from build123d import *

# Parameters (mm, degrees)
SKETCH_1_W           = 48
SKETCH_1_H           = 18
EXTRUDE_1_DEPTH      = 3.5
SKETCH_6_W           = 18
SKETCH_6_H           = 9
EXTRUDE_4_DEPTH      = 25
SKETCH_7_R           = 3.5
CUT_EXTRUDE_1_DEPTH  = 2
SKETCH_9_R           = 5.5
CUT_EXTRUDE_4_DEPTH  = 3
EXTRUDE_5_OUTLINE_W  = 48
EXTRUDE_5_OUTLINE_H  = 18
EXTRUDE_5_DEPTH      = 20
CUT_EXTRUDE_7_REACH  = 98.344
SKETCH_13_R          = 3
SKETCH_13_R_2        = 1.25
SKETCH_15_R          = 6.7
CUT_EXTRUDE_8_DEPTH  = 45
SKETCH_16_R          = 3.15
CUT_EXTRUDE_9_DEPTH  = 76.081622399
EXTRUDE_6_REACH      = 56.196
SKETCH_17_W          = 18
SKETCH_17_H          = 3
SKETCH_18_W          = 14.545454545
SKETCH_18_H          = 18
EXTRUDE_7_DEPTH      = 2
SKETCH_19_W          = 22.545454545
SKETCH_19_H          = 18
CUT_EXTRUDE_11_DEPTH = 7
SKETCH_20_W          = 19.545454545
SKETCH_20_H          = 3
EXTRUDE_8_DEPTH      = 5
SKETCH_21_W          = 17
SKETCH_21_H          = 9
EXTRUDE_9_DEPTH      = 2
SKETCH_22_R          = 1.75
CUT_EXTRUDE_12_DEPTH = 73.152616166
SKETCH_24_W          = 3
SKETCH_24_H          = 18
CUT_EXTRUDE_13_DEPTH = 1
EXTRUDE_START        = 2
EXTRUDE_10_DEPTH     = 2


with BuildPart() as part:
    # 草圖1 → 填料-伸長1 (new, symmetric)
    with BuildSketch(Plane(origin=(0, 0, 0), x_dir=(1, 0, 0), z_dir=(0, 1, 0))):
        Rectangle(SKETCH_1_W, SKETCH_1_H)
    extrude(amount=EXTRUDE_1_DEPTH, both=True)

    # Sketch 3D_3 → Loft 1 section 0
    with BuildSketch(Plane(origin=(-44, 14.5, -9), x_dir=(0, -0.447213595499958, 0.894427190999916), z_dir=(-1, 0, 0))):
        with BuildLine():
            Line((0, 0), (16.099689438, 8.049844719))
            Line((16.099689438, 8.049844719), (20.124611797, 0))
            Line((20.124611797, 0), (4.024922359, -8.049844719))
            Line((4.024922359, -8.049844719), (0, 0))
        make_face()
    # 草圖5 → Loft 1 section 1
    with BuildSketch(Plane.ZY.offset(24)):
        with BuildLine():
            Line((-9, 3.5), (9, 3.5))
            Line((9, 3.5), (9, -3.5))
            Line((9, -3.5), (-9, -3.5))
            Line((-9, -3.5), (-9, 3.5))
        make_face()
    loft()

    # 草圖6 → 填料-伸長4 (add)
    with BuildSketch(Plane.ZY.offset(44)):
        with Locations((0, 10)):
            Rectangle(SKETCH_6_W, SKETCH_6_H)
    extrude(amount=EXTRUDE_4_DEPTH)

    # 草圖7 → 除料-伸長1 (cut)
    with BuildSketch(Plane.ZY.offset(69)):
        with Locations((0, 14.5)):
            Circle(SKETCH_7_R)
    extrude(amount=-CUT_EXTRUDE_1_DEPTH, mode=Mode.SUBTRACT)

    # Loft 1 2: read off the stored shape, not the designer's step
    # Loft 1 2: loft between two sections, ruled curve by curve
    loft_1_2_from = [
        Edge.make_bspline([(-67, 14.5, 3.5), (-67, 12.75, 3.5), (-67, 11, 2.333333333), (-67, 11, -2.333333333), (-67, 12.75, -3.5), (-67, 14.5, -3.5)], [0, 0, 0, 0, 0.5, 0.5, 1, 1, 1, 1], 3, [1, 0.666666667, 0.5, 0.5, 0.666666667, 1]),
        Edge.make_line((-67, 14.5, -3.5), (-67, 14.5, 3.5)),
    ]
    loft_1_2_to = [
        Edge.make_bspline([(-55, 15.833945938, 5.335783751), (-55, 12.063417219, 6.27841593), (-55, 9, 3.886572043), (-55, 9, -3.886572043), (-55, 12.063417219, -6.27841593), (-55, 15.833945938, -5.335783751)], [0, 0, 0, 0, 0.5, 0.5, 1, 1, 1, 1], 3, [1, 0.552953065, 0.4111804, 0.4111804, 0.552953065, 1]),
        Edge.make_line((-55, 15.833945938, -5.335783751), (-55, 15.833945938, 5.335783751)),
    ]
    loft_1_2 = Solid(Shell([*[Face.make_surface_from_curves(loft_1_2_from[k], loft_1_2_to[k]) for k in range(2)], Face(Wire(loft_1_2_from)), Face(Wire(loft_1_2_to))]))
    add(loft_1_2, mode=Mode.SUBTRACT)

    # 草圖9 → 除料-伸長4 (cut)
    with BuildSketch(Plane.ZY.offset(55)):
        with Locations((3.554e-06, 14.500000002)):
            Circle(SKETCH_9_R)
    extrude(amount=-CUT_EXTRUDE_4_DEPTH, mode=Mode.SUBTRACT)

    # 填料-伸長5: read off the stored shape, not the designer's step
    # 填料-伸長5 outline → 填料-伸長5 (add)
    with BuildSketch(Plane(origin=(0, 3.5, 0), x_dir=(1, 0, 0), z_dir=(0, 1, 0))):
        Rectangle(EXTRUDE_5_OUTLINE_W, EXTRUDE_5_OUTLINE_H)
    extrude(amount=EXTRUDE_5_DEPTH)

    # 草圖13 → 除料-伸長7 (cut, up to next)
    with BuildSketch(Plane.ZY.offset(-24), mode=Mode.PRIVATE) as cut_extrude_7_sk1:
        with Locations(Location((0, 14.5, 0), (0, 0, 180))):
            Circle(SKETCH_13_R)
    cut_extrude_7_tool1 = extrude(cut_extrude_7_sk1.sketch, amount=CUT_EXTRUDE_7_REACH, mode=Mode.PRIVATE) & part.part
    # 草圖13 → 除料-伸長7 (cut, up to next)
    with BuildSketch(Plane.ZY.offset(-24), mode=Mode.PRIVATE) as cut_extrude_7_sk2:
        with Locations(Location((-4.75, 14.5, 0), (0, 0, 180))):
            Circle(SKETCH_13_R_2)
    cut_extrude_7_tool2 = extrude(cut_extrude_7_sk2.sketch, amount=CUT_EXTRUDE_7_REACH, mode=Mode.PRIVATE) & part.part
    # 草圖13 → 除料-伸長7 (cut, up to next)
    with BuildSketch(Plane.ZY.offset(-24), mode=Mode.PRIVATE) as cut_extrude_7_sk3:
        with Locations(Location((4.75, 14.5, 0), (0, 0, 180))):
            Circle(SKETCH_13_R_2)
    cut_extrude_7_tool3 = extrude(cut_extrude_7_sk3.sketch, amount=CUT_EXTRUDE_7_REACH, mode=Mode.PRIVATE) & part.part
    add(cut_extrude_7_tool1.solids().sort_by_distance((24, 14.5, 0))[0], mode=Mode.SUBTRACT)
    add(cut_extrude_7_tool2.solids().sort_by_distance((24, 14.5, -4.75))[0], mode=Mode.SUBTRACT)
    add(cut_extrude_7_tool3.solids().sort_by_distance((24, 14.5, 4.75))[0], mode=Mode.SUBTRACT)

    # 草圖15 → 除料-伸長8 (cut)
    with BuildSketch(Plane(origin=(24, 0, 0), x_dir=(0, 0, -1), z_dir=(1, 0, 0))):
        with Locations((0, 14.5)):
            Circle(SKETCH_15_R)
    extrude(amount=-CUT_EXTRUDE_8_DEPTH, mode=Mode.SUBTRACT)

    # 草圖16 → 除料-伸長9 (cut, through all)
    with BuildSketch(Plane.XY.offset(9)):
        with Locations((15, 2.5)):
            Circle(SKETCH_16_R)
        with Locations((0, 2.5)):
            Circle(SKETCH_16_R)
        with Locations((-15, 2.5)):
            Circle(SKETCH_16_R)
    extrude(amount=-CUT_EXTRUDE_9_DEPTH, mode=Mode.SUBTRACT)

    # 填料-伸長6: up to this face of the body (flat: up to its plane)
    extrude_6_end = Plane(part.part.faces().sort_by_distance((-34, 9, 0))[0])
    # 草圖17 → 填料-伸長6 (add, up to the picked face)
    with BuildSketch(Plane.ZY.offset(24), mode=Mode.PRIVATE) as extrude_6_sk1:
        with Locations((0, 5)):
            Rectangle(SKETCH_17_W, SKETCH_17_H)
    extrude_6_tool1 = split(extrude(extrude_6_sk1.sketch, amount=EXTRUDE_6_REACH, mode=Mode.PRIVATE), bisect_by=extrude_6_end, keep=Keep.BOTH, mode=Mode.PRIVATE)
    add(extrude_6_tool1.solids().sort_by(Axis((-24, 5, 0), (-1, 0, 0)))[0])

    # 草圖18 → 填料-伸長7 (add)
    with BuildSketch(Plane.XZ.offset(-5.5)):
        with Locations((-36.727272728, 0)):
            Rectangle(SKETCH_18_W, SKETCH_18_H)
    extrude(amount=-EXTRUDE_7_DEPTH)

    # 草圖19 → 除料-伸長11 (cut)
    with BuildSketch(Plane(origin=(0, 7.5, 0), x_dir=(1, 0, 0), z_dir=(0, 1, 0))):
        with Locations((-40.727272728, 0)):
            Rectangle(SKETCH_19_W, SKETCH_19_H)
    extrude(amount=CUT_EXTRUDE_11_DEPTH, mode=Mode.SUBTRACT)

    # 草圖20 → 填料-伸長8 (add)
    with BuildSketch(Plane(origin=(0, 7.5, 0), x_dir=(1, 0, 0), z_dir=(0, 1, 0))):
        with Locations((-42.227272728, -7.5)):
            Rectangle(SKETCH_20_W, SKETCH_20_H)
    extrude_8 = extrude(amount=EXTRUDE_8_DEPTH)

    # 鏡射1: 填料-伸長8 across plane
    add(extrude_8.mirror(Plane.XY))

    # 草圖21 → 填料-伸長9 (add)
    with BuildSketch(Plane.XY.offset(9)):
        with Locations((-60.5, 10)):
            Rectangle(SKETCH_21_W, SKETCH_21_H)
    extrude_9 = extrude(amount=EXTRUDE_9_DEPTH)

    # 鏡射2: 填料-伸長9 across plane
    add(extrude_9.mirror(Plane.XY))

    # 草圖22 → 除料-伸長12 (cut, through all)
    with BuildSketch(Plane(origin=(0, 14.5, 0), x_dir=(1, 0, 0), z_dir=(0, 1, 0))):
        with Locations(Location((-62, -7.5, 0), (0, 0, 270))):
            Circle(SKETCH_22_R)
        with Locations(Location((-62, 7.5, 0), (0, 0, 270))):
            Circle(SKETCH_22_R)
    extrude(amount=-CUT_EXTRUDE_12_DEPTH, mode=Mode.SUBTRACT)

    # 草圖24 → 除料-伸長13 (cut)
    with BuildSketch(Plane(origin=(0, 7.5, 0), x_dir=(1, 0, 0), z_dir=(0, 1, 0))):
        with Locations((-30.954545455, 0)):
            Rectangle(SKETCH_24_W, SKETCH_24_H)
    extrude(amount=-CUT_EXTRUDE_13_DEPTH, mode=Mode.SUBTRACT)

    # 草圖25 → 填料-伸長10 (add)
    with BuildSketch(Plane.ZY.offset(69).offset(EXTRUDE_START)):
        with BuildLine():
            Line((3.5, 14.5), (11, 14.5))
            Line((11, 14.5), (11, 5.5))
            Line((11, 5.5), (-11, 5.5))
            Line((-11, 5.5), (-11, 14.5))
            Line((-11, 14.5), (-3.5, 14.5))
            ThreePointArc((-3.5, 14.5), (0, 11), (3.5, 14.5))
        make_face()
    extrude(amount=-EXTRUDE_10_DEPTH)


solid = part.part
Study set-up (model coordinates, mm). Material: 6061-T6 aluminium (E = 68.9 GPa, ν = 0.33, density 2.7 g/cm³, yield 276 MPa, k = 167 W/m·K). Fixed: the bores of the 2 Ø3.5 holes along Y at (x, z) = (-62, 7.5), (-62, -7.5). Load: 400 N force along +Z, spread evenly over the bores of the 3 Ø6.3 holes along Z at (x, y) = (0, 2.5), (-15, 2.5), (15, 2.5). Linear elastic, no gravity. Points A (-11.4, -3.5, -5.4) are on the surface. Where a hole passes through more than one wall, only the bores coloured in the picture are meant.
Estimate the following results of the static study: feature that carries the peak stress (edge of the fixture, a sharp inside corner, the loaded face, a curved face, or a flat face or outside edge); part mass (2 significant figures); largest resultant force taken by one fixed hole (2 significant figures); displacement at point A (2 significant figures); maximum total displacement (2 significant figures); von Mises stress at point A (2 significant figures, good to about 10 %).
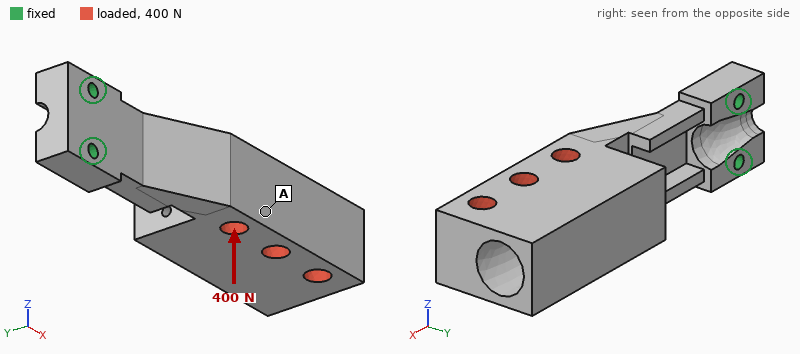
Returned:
a curved face
57 g
1.5 kN
0.10 mm
0.33 mm
9.2 MPa
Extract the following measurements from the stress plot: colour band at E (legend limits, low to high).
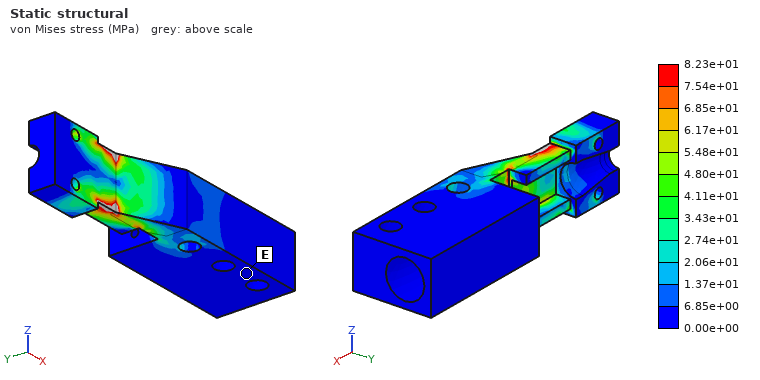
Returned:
0.00e+00 to 6.85e+00 MPa
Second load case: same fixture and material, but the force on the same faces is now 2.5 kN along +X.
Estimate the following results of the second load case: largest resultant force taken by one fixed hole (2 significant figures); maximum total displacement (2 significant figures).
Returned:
1.3 kN
1.0 mm
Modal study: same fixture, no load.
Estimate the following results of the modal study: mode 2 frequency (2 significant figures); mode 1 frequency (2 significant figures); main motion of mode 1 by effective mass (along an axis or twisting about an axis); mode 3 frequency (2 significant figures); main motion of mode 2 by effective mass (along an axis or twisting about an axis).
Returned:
940 Hz
450 Hz
along Y
2400 Hz
along Z
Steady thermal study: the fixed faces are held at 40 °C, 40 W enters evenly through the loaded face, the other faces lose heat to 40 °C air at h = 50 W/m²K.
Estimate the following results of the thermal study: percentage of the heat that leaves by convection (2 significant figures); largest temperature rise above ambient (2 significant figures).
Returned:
53 %
60 K
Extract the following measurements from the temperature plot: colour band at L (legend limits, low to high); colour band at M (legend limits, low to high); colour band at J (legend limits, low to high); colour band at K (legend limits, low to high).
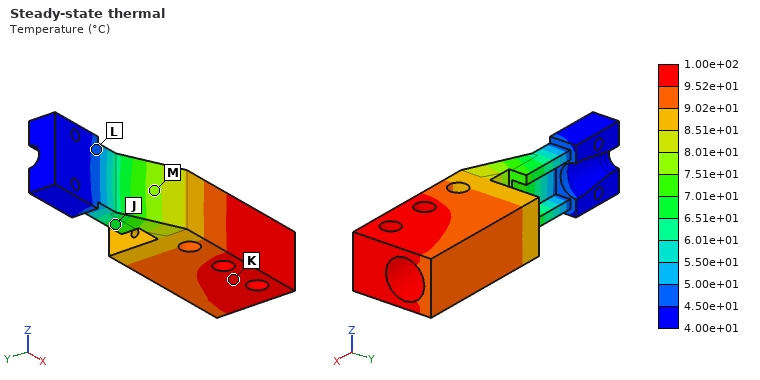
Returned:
4.50e+01 to 5.00e+01 °C
7.51e+01 to 8.01e+01 °C
6.51e+01 to 7.01e+01 °C
9.52e+01 to 1.00e+02 °C
